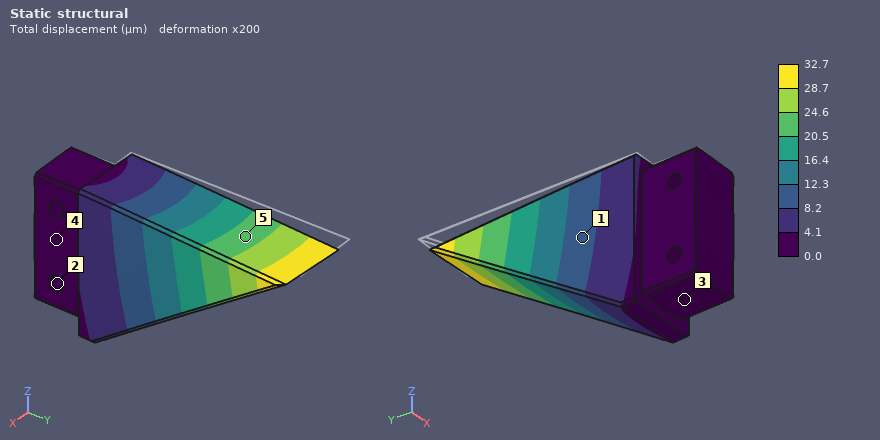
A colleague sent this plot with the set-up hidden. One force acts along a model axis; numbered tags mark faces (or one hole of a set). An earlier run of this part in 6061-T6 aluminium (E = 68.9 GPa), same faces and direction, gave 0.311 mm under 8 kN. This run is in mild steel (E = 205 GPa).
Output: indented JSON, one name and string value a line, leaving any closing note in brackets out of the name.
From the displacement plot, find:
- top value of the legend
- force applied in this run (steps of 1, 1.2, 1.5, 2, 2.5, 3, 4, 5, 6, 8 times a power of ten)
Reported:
{
  "top value of the legend": "32.7 µm",
  "force applied in this run": "2.5 kN"
}
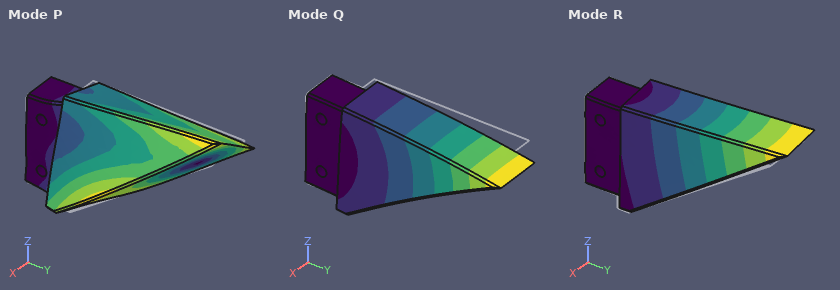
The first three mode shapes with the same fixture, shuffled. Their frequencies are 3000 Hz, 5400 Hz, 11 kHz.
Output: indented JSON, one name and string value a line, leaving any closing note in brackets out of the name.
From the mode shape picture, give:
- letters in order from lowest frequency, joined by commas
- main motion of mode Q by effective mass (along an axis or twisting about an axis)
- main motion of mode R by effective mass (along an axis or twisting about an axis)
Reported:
{
  "letters in order from lowest frequency, joined by commas": "R, Q, P",
  "main motion of mode Q by effective mass": "along Z",
  "main motion of mode R by effective mass": "along X"
}
